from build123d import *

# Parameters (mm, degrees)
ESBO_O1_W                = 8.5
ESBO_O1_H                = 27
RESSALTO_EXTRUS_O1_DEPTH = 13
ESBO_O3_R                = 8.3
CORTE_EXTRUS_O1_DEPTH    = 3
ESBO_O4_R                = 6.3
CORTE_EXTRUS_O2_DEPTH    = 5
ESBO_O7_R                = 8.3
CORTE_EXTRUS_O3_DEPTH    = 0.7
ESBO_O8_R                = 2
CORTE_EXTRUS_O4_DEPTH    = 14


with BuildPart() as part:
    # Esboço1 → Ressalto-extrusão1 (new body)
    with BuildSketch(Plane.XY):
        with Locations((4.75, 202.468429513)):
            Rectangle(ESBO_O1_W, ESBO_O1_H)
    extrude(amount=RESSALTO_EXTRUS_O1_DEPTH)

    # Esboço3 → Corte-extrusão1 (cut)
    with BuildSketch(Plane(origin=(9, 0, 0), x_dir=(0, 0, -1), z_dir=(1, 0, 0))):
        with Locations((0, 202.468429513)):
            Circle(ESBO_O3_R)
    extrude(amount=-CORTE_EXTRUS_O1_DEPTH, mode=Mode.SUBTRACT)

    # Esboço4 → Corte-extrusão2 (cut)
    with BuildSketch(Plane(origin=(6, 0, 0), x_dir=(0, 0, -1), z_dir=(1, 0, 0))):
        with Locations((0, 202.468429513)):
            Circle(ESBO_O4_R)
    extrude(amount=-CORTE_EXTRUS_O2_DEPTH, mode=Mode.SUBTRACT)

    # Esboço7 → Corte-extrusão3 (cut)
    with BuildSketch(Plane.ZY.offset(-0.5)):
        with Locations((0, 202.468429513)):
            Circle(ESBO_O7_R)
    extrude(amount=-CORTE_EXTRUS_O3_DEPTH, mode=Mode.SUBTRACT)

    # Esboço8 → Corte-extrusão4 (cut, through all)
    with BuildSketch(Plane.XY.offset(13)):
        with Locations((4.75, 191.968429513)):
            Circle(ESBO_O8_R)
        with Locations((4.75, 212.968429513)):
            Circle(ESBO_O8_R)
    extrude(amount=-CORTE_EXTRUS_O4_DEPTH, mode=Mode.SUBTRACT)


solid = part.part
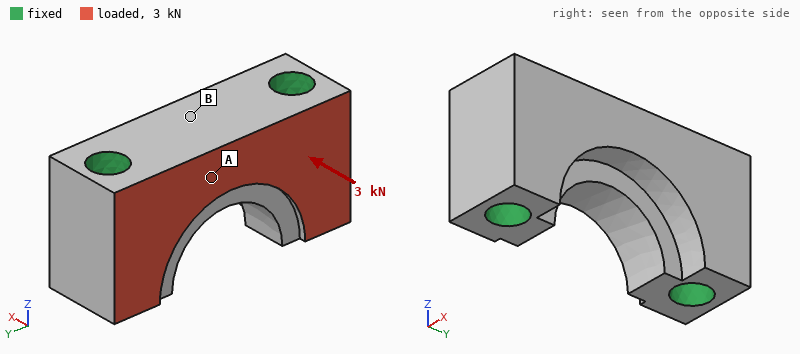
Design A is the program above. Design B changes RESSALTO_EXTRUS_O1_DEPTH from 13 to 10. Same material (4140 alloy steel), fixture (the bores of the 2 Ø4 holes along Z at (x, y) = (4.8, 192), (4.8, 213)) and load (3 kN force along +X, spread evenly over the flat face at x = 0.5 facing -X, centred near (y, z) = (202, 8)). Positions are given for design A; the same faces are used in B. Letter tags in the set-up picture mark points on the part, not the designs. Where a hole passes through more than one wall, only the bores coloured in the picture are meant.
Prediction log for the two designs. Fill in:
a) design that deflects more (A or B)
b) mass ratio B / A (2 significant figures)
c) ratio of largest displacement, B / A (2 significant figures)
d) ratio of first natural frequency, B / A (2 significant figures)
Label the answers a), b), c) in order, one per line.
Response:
a) B
b) 0.69
c) 1.2
d) 1.1
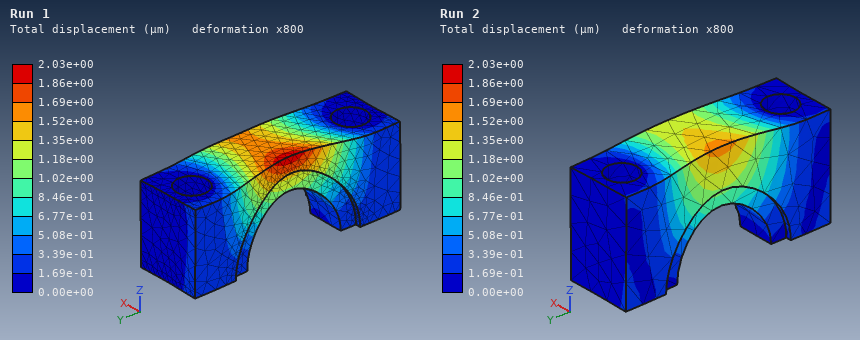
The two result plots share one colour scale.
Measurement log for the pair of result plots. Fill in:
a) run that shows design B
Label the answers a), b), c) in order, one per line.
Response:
a) Run 1
